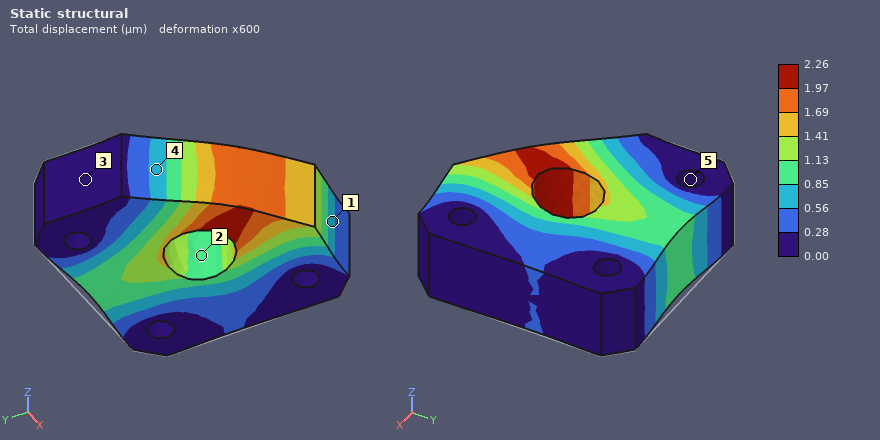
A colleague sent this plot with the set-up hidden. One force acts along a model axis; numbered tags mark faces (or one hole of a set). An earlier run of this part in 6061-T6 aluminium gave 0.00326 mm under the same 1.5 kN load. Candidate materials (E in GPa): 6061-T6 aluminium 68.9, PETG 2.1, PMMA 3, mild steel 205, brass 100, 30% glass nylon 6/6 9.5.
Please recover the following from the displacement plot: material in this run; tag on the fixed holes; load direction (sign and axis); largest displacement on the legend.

brass
5
-Y
2.26 µm
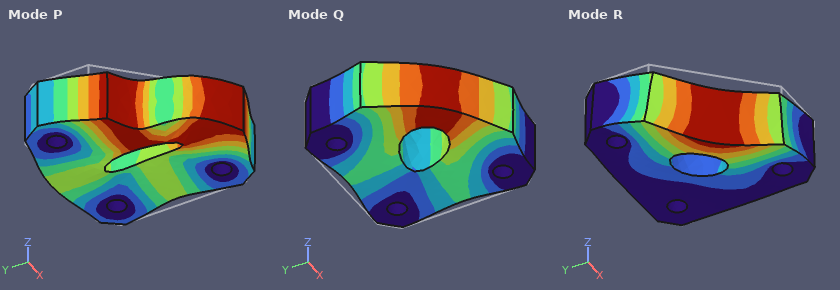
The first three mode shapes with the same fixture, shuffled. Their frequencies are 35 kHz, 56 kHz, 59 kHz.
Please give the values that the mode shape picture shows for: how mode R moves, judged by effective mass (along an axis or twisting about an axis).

along Z
